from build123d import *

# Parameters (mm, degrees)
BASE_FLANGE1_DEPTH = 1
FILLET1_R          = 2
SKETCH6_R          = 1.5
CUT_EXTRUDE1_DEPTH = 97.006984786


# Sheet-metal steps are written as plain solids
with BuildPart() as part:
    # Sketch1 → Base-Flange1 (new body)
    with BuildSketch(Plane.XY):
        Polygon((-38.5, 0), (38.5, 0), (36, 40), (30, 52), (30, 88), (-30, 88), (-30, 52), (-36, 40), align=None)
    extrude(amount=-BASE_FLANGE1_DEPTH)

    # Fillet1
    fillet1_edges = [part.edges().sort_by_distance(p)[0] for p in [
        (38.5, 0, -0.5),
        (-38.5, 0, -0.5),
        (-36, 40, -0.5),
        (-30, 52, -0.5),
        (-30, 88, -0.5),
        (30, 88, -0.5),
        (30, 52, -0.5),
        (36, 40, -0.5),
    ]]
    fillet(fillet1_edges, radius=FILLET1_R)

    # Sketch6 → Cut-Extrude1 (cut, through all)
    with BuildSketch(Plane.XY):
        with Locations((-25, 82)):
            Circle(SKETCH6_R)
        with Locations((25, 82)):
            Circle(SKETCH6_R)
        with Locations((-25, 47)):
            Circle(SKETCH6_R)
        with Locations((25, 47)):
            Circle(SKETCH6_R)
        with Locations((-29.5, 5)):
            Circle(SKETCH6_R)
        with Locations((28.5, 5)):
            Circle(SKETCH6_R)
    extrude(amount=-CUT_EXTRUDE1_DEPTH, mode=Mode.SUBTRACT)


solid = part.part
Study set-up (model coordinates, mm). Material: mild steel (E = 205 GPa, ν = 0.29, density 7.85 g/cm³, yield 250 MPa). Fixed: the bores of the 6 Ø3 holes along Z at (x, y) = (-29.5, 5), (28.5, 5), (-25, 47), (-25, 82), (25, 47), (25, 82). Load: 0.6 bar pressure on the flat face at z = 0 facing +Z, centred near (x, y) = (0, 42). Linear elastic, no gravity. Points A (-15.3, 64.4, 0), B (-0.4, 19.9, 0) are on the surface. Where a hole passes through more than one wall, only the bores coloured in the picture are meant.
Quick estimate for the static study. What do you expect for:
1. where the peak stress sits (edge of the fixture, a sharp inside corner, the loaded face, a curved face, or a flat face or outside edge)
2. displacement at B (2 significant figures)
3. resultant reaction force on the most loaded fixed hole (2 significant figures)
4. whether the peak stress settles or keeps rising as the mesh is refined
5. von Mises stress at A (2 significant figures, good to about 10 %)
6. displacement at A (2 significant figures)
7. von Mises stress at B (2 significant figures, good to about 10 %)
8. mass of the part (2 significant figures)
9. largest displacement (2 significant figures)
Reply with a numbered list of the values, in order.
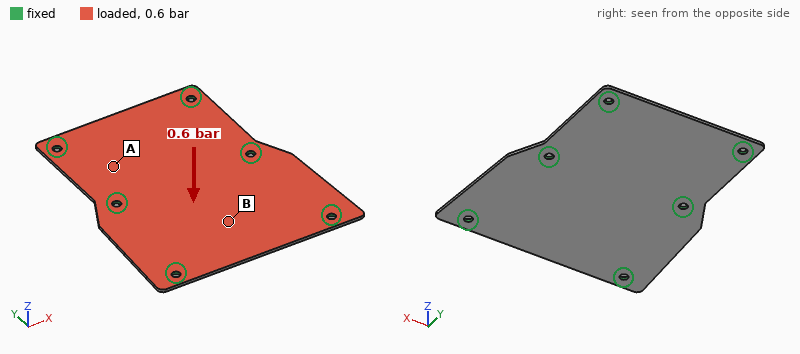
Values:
1. edge of the fixture
2. 0.12 mm
3. 81 N
4. keeps rising
5. 19 MPa
6. 0.044 mm
7. 42 MPa
8. 46 g
9. 0.12 mm
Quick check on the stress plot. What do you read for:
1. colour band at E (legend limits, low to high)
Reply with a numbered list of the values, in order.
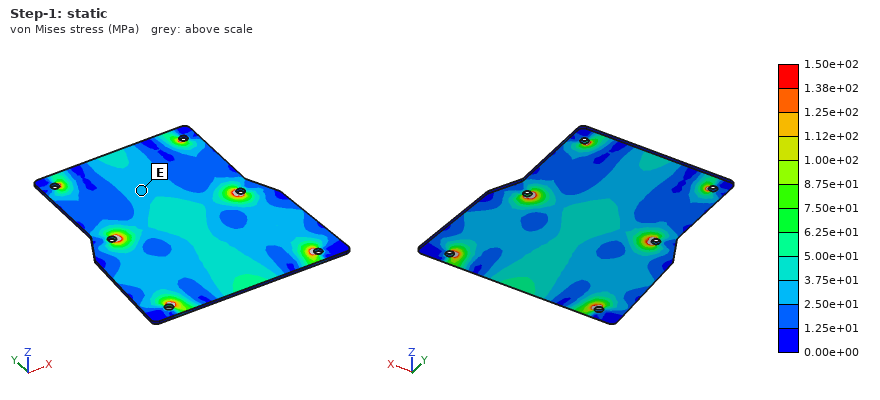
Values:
1. 2.50e+01 to 3.75e+01 MPa
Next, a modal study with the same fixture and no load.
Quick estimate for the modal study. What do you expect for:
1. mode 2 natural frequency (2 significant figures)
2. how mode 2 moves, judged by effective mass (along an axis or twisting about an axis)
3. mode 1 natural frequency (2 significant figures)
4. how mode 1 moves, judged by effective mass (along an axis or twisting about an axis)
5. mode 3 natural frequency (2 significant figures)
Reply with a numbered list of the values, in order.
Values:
1. 1900 Hz
2. along Z
3. 1500 Hz
4. along Z
5. 2500 Hz
